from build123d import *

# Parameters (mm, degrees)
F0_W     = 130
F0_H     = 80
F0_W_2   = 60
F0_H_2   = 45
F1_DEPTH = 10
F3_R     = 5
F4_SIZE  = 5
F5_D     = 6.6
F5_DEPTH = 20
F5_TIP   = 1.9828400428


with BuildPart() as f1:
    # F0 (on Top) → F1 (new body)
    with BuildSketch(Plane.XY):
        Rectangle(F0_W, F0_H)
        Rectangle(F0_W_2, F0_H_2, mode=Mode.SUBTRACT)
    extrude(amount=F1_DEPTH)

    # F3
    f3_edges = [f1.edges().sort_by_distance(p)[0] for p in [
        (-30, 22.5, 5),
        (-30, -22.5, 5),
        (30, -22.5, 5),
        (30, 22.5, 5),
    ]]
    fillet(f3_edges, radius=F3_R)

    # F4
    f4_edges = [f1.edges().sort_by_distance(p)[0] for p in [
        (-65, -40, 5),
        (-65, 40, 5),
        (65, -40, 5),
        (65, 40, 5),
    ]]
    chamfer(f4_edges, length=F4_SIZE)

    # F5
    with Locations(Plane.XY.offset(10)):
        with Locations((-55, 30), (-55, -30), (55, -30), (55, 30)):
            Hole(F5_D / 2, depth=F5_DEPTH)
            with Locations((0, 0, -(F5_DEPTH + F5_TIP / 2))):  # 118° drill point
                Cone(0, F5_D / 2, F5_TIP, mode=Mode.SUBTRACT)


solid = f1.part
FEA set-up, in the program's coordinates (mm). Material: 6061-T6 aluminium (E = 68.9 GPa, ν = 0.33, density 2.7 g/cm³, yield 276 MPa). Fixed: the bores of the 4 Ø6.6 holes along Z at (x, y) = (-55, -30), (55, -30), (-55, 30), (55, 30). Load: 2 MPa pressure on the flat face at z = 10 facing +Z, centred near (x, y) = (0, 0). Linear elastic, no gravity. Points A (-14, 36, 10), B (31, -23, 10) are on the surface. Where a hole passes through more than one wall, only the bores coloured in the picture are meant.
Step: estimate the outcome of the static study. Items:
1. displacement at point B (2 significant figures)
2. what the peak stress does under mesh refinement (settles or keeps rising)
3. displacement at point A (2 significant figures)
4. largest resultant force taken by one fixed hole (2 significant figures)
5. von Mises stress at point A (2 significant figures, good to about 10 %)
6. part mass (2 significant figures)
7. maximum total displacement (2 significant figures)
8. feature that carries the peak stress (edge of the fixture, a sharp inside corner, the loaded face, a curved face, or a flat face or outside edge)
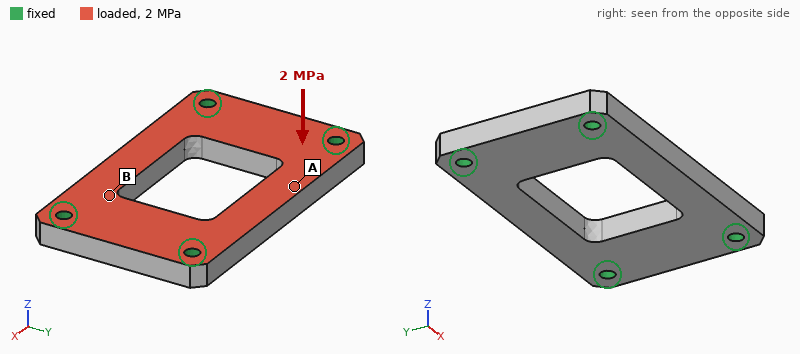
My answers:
0.069 mm
keeps rising
0.11 mm
3.8 kN
43 MPa
200 g
0.14 mm
edge of the fixture
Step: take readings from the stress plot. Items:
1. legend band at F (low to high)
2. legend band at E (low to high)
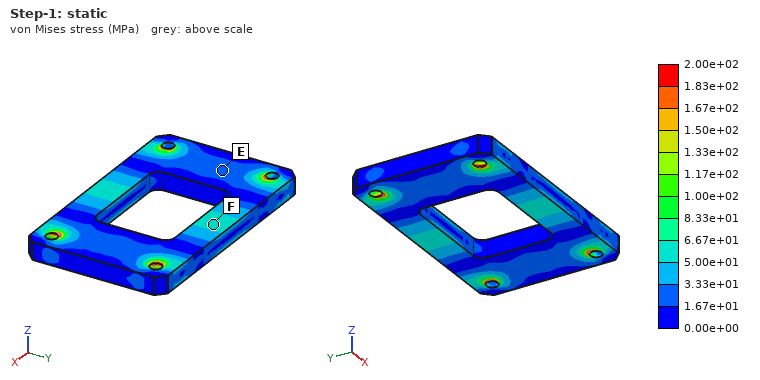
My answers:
5.00e+01 to 6.67e+01 MPa
1.67e+01 to 3.33e+01 MPa
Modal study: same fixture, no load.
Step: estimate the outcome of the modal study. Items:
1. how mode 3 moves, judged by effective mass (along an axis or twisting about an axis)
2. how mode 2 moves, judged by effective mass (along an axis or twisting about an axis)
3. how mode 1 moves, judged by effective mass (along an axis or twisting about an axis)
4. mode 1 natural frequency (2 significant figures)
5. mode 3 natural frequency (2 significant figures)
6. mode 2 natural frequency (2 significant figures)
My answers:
twisting about Y
twisting about X
along Z
4500 Hz
9000 Hz
5000 Hz
